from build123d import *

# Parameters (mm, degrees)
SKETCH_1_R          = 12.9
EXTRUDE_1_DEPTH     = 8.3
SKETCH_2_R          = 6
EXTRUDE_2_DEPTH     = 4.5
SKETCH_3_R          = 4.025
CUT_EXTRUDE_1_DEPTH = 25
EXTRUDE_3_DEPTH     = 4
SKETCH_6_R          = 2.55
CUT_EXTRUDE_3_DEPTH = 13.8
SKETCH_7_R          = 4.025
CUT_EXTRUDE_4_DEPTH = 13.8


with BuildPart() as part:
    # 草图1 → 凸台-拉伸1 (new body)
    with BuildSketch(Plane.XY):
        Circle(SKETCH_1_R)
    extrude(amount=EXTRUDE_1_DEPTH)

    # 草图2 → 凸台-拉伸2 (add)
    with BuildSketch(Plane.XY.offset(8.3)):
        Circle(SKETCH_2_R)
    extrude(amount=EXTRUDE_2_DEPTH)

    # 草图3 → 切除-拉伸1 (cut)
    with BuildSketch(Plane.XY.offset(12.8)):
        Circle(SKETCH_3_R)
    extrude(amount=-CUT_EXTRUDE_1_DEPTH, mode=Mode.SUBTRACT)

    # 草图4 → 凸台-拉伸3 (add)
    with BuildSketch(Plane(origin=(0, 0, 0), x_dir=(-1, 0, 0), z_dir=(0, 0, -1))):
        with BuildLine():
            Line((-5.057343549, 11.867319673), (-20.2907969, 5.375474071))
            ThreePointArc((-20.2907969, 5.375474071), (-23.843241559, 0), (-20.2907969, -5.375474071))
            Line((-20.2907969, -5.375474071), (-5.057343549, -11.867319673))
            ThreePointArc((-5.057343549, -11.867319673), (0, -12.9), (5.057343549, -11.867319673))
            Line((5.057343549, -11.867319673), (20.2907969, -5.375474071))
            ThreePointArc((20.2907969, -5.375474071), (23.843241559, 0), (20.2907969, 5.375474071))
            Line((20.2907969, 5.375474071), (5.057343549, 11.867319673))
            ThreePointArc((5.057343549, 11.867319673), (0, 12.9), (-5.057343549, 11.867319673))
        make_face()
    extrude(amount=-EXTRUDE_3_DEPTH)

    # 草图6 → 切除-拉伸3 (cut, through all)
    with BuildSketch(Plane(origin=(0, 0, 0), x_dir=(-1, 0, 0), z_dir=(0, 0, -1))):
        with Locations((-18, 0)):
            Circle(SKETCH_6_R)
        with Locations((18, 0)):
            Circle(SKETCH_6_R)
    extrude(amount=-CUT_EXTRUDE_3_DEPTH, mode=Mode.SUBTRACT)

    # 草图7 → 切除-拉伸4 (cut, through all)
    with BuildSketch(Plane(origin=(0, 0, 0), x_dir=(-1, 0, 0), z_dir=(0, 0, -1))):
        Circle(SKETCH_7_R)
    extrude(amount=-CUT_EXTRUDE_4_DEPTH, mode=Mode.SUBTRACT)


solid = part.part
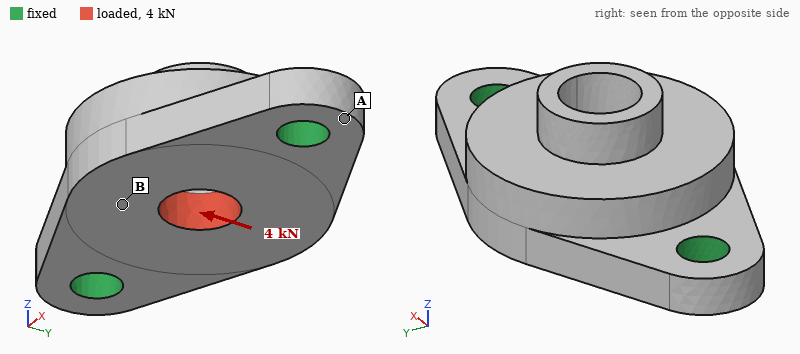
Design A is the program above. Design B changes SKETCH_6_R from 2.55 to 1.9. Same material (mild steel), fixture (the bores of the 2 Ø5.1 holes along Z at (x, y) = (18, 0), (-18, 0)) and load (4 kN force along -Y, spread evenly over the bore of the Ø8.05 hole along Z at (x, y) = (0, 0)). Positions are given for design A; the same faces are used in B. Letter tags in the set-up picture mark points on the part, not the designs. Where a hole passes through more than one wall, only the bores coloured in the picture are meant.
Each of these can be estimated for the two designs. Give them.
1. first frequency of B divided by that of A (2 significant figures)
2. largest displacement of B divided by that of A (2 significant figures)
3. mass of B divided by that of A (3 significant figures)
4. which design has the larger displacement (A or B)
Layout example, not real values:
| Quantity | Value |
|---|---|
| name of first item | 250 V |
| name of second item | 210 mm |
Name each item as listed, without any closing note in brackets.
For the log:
| Quantity | Value |
|---|---|
| first frequency of B divided by that of A | 0.89 |
| largest displacement of B divided by that of A | 1.1 |
| mass of B divided by that of A | 1.01 |
| which design has the larger displacement | B |
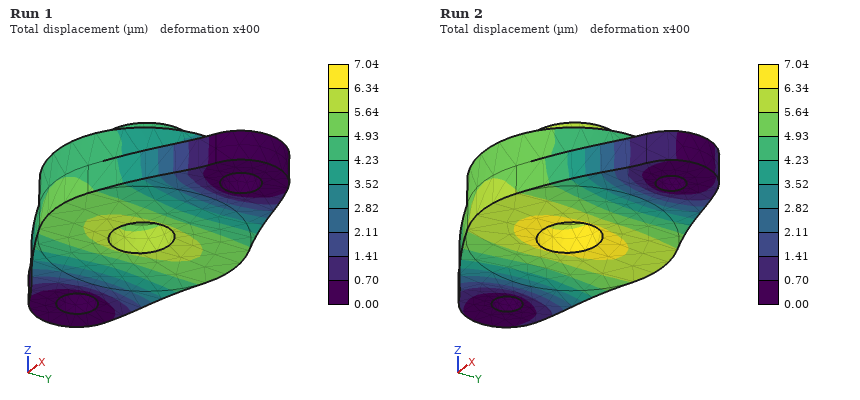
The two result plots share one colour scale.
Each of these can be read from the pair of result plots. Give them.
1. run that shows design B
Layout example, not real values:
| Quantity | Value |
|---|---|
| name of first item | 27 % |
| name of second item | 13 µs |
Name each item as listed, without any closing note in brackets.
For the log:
| Quantity | Value |
|---|---|
| run that shows design B | Run 2 |
